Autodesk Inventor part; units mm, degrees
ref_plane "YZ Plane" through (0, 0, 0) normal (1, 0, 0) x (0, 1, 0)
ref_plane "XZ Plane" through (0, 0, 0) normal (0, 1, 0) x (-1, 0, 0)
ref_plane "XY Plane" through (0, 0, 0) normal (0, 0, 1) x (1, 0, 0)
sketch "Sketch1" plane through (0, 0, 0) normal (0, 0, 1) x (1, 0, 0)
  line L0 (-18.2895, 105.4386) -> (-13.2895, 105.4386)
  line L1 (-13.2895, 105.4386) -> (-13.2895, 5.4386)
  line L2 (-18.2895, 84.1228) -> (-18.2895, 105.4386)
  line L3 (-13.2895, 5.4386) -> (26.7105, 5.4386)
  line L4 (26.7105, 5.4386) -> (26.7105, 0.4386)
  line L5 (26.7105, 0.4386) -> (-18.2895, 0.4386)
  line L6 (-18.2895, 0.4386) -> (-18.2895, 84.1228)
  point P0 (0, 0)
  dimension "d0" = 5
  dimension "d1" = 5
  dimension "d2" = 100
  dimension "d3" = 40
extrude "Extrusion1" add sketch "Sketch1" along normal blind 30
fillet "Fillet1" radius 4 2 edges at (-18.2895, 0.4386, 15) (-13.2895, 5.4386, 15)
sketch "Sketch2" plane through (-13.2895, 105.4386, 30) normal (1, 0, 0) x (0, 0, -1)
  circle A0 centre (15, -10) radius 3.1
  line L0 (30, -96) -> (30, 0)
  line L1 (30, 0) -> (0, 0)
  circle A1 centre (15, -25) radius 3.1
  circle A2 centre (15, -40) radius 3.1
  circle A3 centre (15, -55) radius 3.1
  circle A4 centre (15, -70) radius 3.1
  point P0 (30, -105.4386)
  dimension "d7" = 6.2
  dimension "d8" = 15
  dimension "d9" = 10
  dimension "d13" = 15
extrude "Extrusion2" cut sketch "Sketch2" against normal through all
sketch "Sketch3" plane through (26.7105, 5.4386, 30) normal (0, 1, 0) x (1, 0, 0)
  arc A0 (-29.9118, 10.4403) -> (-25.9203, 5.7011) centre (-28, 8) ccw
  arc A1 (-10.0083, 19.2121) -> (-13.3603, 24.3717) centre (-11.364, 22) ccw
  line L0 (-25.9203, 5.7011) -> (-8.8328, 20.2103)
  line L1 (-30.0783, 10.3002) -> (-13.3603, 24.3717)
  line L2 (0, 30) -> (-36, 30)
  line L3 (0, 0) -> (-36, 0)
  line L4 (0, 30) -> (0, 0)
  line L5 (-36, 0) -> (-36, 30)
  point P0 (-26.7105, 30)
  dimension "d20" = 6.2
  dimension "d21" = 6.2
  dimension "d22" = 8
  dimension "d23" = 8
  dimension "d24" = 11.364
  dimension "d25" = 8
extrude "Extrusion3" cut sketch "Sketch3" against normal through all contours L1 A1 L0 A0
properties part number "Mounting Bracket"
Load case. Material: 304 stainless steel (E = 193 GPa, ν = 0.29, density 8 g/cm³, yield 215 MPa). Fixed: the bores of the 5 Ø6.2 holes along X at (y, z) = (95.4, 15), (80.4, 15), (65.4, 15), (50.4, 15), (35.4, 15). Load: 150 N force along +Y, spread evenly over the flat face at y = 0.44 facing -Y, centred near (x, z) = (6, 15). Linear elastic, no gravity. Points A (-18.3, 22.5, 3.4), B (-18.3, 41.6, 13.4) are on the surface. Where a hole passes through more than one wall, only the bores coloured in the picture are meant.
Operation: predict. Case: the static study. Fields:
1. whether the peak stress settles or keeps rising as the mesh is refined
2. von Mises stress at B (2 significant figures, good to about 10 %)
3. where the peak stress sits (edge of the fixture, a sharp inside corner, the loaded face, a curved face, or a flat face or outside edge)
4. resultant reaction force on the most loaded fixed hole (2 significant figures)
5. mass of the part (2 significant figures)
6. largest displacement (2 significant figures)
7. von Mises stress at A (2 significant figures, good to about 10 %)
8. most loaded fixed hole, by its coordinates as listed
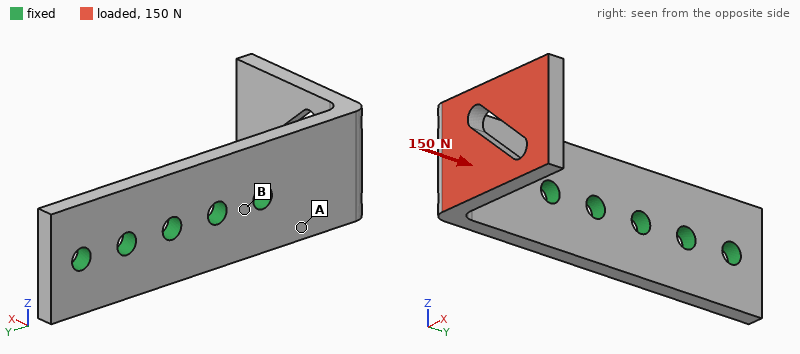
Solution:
keeps rising
4.1 MPa
edge of the fixture
130 N
160 g
0.10 mm
25 MPa
(35.4, 15)
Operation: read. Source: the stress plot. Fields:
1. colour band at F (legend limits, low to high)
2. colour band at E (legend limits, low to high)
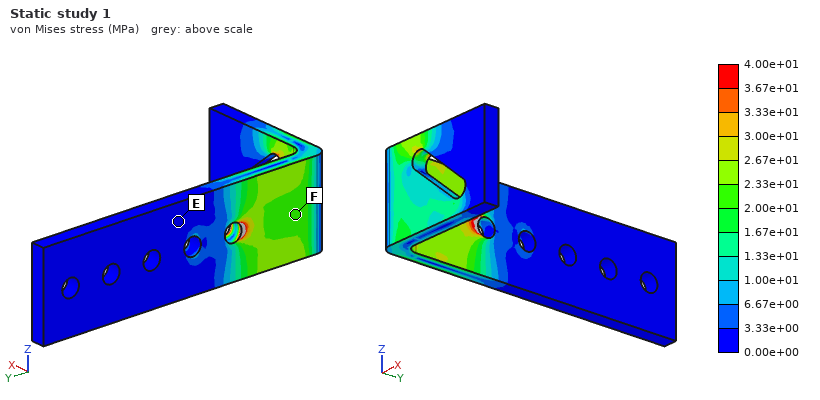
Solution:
2.00e+01 to 2.33e+01 MPa
0.00e+00 to 3.33e+00 MPa
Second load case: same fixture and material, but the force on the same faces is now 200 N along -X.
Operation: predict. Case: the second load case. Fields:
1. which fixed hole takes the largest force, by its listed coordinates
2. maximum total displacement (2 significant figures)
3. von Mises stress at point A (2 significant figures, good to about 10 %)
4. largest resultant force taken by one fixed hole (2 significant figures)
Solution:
(35.4, 15)
98 µm
34 MPa
330 N
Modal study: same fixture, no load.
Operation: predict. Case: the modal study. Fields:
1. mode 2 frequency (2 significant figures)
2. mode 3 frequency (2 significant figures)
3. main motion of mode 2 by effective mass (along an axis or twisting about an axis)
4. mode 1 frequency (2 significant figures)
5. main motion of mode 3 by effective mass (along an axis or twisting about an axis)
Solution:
1600 Hz
2800 Hz
along Z
1000 Hz
along X
